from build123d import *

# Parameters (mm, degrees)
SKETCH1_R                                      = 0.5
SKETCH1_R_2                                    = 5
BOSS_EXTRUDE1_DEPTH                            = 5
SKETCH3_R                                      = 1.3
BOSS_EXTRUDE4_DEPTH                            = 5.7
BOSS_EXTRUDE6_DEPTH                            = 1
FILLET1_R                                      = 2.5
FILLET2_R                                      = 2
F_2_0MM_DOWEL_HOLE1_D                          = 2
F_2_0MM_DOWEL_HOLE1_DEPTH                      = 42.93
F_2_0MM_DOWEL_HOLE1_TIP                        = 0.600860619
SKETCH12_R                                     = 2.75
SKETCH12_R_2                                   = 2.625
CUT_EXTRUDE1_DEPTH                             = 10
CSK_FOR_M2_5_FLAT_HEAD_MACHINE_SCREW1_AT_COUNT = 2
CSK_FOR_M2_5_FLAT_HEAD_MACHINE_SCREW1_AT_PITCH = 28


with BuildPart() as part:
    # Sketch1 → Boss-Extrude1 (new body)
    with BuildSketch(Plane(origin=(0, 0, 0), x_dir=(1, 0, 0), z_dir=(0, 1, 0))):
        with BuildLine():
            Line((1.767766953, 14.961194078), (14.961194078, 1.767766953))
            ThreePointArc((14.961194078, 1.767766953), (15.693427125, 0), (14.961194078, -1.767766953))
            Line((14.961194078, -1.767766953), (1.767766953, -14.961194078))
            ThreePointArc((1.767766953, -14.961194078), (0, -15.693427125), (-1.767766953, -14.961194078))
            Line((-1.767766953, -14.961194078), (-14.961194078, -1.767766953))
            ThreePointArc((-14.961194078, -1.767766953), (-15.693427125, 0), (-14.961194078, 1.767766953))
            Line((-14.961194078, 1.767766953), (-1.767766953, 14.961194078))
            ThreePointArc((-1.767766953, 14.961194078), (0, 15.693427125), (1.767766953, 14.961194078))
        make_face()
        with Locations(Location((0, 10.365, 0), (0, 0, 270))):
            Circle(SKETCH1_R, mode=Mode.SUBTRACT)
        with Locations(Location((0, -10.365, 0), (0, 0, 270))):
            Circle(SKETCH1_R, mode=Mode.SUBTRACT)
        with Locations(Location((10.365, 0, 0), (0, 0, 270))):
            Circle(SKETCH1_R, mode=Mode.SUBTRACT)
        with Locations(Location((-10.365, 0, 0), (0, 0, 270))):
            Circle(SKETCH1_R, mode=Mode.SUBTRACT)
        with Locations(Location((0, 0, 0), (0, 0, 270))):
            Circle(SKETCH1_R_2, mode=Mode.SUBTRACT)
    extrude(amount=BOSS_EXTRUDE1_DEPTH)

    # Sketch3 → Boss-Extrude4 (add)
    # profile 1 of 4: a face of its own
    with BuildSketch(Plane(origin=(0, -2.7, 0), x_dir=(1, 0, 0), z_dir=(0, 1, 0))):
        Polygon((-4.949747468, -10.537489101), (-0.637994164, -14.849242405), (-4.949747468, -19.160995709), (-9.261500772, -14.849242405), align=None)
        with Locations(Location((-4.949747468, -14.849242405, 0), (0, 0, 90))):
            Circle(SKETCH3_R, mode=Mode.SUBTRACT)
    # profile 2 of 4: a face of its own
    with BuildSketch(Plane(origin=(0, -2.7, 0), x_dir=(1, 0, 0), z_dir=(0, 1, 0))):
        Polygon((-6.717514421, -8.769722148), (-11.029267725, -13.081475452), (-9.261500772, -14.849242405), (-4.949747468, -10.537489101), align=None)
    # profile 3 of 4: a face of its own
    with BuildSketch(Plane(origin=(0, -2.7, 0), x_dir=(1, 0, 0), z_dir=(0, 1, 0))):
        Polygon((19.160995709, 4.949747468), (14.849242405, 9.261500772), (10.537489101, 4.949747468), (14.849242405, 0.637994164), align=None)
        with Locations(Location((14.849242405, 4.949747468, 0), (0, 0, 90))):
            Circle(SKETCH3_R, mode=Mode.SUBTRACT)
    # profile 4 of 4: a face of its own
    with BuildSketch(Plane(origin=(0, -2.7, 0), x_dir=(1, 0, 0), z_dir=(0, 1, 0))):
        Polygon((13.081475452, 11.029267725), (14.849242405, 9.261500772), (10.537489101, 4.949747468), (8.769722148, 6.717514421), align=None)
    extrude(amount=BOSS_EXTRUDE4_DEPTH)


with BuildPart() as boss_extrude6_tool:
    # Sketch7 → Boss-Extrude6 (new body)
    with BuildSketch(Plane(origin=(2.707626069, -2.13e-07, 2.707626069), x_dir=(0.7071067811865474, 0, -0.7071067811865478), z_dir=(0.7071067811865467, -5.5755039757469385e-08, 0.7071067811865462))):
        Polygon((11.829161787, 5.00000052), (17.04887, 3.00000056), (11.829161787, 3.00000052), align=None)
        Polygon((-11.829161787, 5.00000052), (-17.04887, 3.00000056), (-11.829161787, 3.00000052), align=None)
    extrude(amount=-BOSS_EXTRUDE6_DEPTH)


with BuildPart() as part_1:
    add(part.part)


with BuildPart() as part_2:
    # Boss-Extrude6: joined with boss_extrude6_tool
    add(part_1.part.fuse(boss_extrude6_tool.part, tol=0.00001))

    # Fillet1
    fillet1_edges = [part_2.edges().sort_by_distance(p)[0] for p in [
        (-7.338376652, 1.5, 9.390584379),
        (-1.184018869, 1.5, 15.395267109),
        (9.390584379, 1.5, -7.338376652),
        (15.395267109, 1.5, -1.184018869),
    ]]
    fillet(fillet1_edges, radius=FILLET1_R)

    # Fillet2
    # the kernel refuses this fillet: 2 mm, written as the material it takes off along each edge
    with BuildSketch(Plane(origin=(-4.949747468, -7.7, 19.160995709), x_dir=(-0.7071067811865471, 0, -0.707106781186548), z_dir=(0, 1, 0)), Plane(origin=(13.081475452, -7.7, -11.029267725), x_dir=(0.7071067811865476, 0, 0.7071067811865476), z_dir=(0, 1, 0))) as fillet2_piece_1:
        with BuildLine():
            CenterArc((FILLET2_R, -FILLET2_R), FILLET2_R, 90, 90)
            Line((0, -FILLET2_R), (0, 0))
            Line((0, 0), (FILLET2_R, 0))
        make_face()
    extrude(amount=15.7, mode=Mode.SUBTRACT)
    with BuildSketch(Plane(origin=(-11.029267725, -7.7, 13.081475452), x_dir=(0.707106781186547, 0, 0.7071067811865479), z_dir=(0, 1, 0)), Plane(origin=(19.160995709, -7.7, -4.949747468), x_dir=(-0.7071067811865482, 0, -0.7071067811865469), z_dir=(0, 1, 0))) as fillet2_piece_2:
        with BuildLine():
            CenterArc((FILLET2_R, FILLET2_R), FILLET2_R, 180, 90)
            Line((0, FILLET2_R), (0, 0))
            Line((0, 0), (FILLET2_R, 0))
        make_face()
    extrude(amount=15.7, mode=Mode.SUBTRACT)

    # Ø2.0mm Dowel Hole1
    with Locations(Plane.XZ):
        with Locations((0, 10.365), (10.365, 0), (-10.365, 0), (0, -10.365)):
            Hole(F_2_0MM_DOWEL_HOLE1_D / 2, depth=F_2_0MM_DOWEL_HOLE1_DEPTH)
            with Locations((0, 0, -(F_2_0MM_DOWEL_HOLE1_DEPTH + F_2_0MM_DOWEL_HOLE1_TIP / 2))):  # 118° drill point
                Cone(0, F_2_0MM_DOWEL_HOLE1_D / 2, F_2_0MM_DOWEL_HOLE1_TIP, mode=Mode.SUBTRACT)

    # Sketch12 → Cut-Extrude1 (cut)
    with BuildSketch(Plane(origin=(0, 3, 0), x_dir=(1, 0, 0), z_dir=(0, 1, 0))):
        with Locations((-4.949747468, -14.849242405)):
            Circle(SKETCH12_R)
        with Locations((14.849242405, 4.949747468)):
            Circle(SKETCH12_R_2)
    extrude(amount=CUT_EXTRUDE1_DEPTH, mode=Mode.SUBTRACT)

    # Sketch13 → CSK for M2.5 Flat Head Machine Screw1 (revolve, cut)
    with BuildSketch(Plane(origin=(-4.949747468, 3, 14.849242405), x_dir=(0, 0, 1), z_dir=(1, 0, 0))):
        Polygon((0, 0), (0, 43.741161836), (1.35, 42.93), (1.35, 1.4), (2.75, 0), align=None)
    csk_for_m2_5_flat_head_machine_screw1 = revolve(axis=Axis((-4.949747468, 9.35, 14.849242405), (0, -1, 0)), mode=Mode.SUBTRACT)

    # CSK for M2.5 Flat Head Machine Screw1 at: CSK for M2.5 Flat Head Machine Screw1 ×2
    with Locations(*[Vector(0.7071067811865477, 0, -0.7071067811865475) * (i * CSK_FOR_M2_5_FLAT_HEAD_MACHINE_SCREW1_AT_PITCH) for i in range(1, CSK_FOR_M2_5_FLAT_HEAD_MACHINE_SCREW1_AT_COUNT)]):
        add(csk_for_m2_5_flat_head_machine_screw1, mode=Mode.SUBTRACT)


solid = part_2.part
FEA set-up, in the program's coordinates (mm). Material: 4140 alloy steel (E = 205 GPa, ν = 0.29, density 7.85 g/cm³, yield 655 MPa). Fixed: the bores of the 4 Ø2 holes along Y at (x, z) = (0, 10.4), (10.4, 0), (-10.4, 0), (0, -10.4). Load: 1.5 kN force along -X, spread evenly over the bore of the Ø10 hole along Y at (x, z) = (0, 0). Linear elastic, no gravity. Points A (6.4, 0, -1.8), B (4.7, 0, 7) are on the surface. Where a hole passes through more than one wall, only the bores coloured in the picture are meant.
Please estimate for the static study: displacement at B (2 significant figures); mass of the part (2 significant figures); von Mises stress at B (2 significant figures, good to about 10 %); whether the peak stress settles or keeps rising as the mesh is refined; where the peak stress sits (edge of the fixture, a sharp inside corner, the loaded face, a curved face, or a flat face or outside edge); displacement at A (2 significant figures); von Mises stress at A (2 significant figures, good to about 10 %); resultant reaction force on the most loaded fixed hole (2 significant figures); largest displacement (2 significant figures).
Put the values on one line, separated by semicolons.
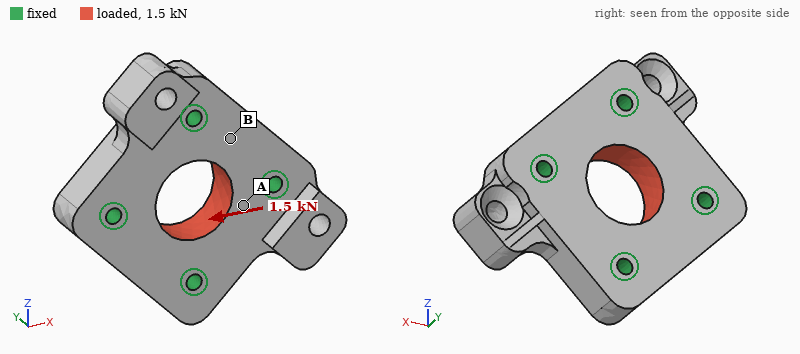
0.36 µm; 22 g; 5.2 MPa; keeps rising; edge of the fixture; 0.30 µm; 14 MPa; 460 N; 0.56 µm
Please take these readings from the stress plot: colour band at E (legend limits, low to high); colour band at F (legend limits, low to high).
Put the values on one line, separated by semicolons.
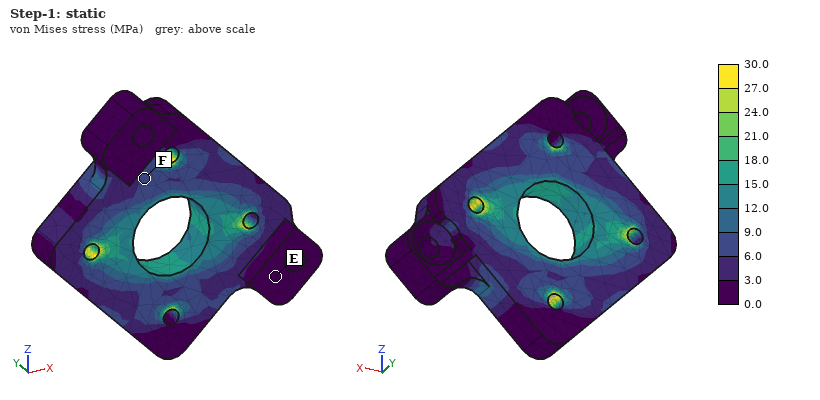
0.0 to 3.0 MPa; 6.0 to 9.0 MPa
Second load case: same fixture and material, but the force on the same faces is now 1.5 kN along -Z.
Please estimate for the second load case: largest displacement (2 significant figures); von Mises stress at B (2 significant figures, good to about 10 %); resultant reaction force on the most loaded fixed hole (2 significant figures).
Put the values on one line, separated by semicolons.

0.56 µm; 7.9 MPa; 460 N
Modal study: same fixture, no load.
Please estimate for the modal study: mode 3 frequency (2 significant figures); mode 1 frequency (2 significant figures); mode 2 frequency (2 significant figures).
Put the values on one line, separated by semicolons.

52 kHz; 31 kHz; 31 kHz
